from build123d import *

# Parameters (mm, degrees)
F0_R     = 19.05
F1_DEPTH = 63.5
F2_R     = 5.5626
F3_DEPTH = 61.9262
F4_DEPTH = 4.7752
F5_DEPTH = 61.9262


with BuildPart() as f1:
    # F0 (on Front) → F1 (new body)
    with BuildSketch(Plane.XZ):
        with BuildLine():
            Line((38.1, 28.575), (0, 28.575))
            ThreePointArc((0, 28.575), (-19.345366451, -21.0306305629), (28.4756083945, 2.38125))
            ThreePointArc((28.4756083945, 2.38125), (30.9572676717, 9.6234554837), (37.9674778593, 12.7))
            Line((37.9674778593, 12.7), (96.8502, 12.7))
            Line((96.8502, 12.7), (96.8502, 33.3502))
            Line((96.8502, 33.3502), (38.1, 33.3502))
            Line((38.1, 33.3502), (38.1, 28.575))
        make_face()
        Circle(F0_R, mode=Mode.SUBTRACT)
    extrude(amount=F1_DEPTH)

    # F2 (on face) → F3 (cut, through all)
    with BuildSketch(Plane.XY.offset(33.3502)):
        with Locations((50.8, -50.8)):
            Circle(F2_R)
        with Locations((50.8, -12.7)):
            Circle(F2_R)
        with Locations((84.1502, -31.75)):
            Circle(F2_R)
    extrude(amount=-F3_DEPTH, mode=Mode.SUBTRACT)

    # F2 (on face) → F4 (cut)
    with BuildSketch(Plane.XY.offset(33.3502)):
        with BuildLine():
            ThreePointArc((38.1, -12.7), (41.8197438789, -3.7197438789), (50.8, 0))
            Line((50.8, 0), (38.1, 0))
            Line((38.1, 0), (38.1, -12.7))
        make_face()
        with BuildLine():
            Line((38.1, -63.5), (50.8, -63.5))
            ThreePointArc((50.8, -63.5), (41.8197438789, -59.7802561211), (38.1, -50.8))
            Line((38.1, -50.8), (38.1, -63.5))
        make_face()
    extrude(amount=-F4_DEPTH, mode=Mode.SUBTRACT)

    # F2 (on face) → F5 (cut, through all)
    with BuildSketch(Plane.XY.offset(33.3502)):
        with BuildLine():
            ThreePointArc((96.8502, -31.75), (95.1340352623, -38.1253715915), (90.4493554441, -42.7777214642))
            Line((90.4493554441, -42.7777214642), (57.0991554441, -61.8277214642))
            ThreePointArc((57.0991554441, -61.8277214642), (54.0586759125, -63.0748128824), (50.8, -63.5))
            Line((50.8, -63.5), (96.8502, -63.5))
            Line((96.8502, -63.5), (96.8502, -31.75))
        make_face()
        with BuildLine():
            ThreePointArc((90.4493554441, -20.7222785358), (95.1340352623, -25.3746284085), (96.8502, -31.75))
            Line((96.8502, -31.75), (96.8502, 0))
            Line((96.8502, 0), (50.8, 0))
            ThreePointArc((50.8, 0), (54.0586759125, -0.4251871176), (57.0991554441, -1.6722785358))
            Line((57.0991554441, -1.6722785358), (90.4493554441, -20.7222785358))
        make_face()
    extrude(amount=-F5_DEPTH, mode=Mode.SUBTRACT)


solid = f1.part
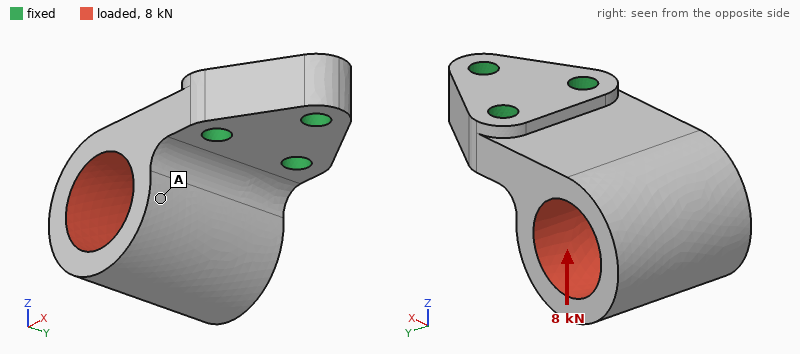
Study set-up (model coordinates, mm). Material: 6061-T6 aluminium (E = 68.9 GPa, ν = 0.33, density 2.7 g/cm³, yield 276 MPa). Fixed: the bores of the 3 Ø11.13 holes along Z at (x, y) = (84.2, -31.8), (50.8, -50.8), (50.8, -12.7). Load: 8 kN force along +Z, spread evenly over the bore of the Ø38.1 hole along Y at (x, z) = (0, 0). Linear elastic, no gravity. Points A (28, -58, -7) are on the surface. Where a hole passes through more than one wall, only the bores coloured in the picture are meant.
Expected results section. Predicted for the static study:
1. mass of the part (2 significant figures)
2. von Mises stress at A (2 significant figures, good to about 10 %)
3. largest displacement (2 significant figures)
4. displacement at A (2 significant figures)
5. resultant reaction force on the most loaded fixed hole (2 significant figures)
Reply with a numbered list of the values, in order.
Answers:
1. 440 g
2. 20 MPa
3. 0.35 mm
4. 0.12 mm
5. 4.7 kN
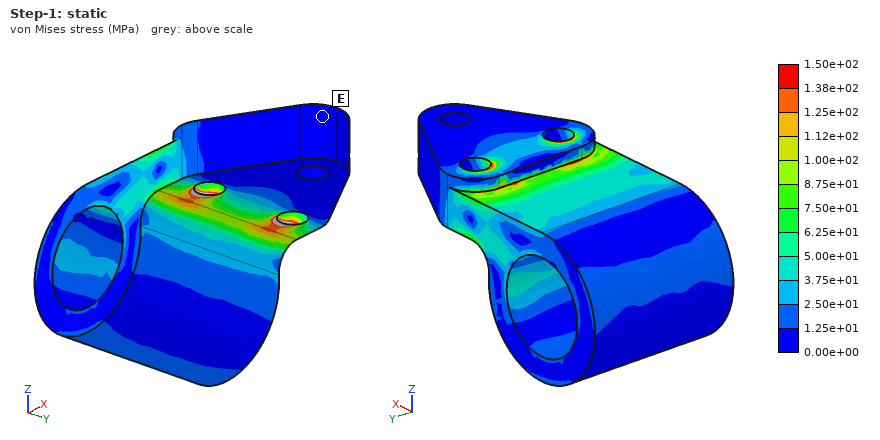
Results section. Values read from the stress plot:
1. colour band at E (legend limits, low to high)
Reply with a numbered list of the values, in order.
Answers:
1. 0.00e+00 to 1.25e+01 MPa
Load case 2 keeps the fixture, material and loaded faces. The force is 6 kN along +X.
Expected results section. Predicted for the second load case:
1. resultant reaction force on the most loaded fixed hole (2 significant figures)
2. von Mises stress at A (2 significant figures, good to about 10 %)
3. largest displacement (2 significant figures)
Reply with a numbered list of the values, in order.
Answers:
1. 2.9 kN
2. 12 MPa
3. 0.16 mm
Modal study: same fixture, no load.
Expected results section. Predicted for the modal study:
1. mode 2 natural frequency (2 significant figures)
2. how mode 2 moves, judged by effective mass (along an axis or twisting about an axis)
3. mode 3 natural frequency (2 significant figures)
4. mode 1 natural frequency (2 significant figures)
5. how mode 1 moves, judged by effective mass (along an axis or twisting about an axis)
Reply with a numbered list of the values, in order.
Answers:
1. 3700 Hz
2. along Y
3. 5900 Hz
4. 1600 Hz
5. along Z
